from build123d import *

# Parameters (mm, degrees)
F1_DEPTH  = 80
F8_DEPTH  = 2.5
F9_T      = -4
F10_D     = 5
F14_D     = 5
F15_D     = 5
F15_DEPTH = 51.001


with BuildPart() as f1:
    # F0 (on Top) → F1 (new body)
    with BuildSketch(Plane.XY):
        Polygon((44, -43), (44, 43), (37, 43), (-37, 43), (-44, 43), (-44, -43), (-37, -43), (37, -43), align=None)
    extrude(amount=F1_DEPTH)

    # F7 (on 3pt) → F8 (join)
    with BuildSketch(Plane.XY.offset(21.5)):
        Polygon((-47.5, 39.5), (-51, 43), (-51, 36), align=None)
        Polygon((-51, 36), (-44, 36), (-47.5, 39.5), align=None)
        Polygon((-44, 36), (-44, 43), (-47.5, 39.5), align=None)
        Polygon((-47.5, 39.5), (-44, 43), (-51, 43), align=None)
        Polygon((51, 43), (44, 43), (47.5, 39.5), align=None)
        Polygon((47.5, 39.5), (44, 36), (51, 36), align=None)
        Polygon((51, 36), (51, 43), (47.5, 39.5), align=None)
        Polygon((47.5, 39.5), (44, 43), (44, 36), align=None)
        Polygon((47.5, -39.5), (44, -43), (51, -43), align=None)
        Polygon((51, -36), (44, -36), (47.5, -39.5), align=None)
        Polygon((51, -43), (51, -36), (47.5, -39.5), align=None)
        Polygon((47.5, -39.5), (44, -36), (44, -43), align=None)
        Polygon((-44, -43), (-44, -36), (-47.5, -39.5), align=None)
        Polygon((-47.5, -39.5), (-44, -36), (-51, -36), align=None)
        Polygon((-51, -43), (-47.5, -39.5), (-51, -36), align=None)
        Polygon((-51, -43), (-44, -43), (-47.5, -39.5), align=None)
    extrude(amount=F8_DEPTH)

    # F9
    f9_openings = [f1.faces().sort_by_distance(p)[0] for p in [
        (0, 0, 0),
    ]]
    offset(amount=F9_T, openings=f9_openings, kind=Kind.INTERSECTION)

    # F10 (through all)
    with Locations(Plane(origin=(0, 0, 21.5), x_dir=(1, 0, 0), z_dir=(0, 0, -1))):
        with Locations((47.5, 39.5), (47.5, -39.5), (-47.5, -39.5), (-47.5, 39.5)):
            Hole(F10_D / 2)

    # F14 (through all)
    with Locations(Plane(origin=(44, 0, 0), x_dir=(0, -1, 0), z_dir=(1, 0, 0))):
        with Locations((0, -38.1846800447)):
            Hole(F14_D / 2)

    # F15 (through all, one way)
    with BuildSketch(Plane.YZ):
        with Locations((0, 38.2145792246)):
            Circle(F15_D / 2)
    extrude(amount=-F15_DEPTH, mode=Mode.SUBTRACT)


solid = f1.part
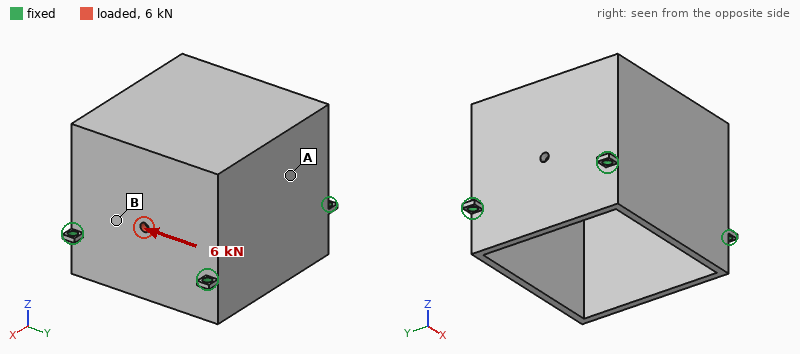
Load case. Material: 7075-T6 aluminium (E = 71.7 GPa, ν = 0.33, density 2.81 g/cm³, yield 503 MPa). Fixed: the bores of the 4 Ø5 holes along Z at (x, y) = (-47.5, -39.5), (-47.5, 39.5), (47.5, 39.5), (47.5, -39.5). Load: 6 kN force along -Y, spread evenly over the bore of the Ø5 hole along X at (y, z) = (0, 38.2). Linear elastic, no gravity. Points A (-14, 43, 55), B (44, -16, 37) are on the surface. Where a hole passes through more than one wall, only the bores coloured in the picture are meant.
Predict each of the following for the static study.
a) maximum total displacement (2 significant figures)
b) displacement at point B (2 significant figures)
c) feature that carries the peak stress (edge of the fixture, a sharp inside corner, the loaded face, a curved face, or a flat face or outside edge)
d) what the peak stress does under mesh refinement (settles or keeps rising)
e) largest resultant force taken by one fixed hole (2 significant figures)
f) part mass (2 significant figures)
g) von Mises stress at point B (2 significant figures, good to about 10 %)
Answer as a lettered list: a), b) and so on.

a) 50 µm
b) 39 µm
c) edge of the fixture
d) keeps rising
e) 2.8 kN
f) 370 g
g) 36 MPa
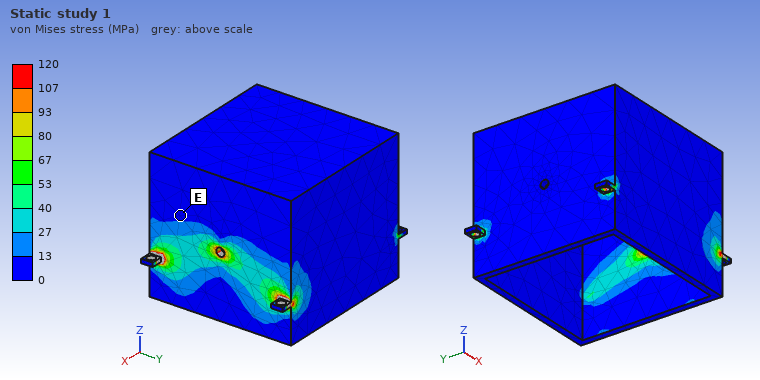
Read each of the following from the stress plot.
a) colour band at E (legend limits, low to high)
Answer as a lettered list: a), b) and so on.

a) 0 to 13 MPa
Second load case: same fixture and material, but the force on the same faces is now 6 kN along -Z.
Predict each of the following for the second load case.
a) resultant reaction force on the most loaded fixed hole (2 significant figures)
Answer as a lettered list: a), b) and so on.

a) 2.9 kN
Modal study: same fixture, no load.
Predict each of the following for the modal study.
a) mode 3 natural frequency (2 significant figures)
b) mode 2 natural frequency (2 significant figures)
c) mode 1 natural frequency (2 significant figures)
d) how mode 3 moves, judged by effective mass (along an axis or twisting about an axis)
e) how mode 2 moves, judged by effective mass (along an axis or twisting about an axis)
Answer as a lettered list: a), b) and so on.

a) 2900 Hz
b) 2400 Hz
c) 2300 Hz
d) along X
e) along Y
